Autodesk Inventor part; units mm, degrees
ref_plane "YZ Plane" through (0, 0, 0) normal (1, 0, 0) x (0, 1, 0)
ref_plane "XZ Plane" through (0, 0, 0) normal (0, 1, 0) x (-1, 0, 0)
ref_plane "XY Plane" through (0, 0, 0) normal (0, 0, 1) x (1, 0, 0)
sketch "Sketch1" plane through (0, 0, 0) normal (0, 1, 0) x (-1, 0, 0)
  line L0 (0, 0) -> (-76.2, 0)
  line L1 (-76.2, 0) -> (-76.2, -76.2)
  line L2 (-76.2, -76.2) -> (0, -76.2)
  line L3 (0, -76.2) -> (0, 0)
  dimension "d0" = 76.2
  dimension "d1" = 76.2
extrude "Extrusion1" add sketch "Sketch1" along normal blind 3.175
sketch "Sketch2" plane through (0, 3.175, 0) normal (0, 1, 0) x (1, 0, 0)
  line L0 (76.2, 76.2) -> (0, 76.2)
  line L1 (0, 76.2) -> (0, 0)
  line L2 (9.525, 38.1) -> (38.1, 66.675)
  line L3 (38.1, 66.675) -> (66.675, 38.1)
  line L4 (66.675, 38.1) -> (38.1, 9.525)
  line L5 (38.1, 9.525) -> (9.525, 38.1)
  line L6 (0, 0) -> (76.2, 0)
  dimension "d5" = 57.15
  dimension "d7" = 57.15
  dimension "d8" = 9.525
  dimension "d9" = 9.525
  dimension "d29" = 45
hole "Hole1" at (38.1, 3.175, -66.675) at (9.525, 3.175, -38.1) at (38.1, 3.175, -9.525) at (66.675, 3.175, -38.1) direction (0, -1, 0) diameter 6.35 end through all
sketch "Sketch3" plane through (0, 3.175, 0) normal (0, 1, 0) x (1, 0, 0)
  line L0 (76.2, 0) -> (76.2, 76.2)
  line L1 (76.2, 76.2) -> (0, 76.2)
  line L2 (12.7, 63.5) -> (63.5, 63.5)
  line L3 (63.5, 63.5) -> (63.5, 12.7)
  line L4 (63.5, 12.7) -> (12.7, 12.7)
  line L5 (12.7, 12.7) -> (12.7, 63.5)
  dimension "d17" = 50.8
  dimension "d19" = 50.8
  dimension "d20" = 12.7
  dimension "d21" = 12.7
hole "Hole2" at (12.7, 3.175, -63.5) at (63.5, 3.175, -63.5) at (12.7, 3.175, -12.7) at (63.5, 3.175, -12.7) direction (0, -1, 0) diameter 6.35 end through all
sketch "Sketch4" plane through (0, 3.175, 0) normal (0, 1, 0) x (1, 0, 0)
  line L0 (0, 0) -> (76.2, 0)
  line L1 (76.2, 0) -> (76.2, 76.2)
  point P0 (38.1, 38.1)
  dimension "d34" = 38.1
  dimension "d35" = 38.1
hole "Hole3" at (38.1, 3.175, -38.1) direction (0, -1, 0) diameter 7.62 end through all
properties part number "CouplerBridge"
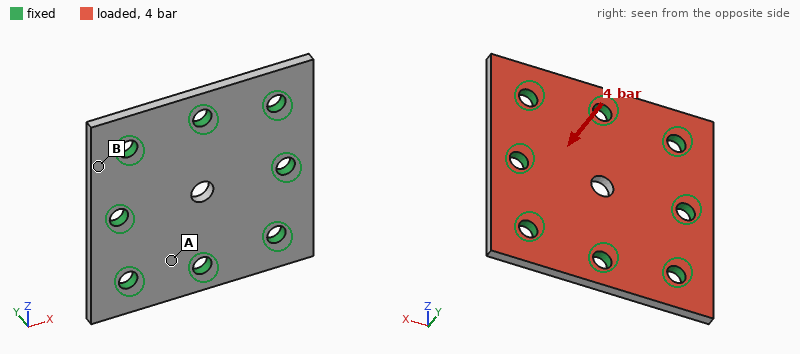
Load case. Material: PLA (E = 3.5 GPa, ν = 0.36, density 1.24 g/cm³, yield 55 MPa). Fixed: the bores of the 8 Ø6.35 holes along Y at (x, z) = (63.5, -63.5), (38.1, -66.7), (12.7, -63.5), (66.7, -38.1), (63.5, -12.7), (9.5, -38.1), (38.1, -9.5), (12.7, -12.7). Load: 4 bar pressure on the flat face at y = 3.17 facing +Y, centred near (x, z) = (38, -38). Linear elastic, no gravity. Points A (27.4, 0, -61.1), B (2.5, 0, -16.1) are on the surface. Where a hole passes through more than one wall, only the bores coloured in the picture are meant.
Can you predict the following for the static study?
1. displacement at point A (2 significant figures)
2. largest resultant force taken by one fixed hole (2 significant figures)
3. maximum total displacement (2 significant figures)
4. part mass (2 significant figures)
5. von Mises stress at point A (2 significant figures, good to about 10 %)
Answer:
0.077 mm
300 N
0.48 mm
22 g
11 MPa
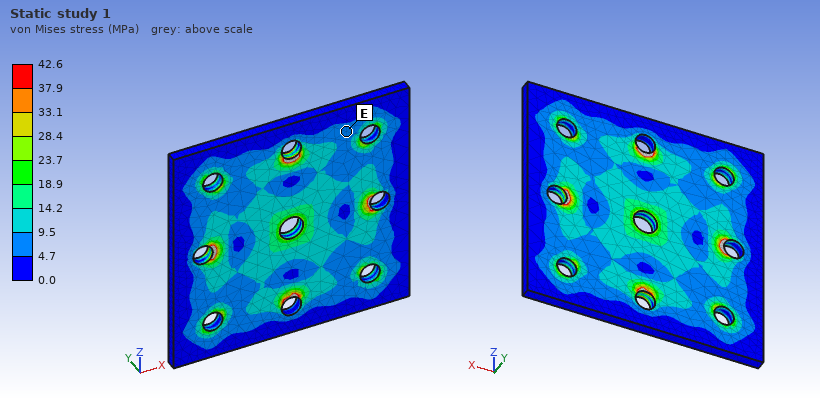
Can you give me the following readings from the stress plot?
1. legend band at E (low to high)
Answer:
4.7 to 9.5 MPa
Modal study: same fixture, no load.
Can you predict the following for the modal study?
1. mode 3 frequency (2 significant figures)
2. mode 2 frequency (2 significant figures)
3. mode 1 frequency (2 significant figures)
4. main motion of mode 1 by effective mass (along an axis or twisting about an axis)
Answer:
5600 Hz
5500 Hz
3000 Hz
along Y
